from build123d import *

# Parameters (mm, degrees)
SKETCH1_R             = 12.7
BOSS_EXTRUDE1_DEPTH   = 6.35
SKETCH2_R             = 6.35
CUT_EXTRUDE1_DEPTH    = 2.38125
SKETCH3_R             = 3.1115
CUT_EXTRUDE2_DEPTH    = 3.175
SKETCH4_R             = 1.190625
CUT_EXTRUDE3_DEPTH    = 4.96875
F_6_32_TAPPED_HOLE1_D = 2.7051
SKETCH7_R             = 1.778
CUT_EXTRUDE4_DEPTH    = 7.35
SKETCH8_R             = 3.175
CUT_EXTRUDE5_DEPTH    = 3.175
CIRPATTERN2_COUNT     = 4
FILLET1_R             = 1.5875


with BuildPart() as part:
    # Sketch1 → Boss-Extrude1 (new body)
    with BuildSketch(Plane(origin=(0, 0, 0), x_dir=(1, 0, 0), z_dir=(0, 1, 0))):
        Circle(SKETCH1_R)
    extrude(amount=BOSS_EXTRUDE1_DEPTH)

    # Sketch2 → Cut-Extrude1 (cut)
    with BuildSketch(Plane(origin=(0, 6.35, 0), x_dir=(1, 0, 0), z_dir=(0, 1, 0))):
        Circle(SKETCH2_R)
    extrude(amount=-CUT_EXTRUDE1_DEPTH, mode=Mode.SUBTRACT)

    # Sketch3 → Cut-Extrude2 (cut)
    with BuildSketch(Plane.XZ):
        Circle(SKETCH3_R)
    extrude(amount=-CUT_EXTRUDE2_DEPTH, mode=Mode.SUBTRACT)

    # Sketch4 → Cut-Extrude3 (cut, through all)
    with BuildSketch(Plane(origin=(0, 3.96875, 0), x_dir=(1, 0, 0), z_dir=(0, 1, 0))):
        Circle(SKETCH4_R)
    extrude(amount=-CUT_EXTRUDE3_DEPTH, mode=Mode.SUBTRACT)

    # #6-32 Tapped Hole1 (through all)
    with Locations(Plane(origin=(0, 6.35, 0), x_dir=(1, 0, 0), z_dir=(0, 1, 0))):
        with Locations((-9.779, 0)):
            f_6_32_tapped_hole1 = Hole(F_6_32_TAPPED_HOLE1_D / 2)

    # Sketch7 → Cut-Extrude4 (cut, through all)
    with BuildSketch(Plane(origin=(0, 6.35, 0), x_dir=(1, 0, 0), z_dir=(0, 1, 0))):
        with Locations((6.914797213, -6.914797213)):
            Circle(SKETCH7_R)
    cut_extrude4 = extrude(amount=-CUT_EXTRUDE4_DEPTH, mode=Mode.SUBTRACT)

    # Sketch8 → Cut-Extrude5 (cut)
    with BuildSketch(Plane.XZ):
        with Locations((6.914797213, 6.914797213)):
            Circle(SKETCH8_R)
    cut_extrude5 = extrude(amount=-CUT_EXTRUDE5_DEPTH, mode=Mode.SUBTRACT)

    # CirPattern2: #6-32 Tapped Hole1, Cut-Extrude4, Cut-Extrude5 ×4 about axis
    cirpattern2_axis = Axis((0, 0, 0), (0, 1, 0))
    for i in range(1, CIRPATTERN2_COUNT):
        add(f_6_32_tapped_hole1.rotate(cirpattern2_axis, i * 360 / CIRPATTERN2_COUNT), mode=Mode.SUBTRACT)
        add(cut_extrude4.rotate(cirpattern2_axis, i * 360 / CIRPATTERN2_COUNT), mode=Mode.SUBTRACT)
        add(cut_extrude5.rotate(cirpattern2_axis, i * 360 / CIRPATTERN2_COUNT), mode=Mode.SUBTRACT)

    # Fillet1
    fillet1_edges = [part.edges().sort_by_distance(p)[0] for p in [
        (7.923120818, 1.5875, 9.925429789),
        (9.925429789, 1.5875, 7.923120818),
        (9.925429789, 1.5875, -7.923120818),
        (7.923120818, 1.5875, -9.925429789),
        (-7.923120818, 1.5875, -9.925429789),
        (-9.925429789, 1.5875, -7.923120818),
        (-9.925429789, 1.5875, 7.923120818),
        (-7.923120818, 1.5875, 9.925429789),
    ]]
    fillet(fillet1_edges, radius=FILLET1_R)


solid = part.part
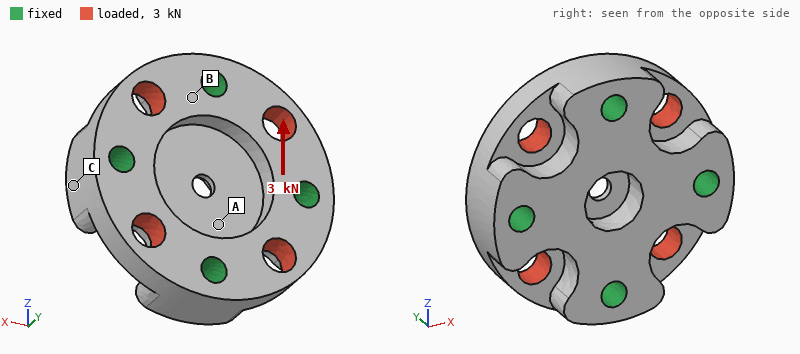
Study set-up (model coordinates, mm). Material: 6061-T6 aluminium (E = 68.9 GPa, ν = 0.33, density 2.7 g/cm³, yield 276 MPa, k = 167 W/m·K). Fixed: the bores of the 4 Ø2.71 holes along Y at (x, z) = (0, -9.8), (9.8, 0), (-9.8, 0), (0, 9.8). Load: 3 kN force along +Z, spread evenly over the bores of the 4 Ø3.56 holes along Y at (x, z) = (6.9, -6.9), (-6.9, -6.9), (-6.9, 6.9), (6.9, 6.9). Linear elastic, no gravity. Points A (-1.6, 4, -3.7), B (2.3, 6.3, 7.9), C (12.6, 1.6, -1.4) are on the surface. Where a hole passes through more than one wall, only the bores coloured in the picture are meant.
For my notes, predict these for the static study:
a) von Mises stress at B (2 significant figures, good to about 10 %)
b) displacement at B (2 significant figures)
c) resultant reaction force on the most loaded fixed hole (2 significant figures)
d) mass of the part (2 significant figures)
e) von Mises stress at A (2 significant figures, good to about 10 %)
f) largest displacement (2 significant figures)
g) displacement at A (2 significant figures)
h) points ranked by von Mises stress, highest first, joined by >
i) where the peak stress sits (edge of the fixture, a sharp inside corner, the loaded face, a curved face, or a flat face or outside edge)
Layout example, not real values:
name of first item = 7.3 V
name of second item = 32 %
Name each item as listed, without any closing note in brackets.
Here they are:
von Mises stress at B = 24 MPa
displacement at B = 1.0 µm
resultant reaction force on the most loaded fixed hole = 910 N
mass of the part = 5.6 g
von Mises stress at A = 14 MPa
largest displacement = 5.1 µm
displacement at A = 1.0 µm
points ranked by von Mises stress, highest first, joined by > = B > A > C
where the peak stress sits = the loaded face
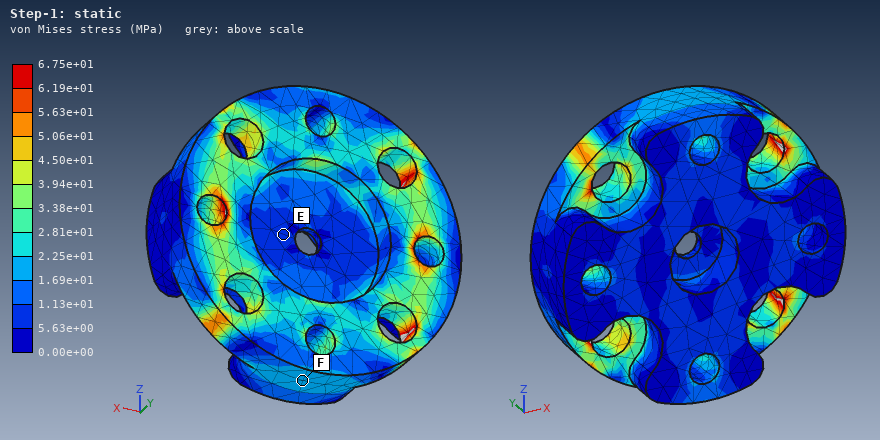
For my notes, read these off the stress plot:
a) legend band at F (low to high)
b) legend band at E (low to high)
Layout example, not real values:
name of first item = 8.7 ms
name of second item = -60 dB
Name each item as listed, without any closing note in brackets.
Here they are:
legend band at F = 1.69e+01 to 2.25e+01 MPa
legend band at E = 5.63e+00 to 1.13e+01 MPa
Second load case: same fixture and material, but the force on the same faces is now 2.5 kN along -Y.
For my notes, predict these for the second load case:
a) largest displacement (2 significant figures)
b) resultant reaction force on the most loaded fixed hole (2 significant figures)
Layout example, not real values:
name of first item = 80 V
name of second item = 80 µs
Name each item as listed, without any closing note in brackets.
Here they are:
largest displacement = 8.7 µm
resultant reaction force on the most loaded fixed hole = 630 N
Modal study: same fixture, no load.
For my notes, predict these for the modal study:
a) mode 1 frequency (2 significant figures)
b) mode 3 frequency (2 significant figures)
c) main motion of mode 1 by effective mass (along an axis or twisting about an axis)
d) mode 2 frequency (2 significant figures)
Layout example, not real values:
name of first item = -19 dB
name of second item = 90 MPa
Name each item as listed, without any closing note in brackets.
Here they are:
mode 1 frequency = 88 kHz
mode 3 frequency = 95 kHz
main motion of mode 1 by effective mass = along Y
mode 2 frequency = 92 kHz
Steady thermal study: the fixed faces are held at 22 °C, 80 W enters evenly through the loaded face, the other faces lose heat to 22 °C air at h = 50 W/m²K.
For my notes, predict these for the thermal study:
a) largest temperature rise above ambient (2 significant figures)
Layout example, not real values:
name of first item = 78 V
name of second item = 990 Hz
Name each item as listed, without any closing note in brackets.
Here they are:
largest temperature rise above ambient = 19 K
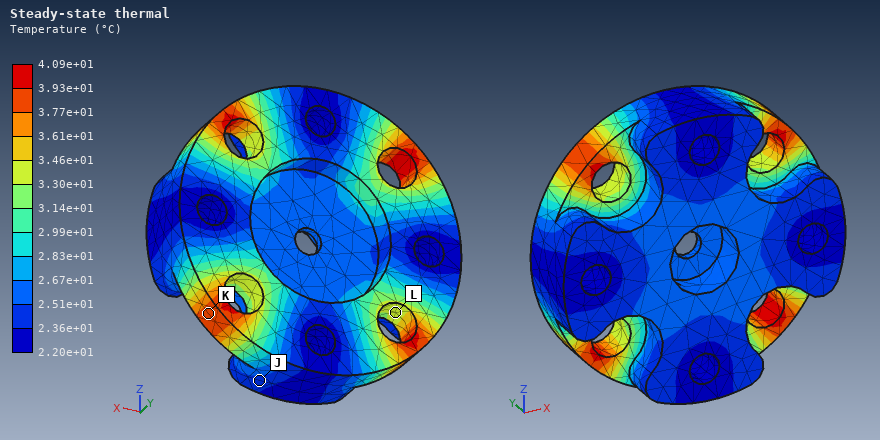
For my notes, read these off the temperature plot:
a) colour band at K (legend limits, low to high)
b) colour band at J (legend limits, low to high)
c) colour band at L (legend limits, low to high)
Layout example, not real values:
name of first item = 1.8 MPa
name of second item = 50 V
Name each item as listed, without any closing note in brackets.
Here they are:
colour band at K = 3.77e+01 to 3.93e+01 °C
colour band at J = 2.36e+01 to 2.51e+01 °C
colour band at L = 3.30e+01 to 3.46e+01 °C
